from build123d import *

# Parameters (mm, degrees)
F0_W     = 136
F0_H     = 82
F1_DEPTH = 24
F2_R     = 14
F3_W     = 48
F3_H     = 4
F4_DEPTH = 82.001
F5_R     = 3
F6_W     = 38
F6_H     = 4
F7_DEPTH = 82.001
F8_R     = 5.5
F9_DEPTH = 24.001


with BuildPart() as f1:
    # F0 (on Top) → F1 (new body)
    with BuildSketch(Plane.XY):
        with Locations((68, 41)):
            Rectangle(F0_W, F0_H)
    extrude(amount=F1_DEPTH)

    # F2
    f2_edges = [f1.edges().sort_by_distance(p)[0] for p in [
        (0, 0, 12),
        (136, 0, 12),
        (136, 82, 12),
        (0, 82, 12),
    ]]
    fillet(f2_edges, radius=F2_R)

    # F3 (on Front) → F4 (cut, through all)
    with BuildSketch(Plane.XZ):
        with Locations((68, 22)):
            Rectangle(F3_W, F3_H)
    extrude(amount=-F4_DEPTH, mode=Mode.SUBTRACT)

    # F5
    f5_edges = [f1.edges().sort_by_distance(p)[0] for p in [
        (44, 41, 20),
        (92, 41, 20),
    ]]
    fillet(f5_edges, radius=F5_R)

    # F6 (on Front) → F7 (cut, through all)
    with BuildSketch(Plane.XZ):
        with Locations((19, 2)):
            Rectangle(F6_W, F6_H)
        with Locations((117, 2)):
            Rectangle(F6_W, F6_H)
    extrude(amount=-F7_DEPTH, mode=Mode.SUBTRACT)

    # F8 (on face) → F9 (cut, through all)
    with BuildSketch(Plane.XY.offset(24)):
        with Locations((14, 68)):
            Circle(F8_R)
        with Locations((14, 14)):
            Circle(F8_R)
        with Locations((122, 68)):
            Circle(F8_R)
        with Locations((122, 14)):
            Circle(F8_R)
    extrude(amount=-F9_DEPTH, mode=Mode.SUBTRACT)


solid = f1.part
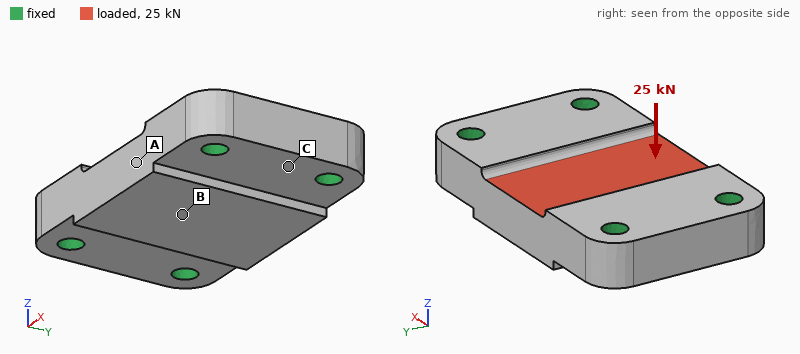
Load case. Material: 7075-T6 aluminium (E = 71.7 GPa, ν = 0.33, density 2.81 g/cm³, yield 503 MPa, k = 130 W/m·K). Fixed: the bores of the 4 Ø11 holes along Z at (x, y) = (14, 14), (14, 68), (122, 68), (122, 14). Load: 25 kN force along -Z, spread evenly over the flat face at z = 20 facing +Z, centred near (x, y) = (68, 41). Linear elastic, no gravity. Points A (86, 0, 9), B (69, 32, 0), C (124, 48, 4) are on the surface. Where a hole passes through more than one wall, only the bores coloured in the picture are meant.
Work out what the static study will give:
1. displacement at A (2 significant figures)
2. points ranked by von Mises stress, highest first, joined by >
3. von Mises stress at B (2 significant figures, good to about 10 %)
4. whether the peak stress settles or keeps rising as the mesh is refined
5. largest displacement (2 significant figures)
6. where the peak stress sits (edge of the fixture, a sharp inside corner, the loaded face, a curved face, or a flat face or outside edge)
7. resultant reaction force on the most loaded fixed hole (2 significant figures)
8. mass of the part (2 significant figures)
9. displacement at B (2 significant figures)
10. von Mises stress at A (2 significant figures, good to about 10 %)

40 µm
B > A > C
39 MPa
keeps rising
51 µm
edge of the fixture
7.2 kN
610 g
46 µm
26 MPa
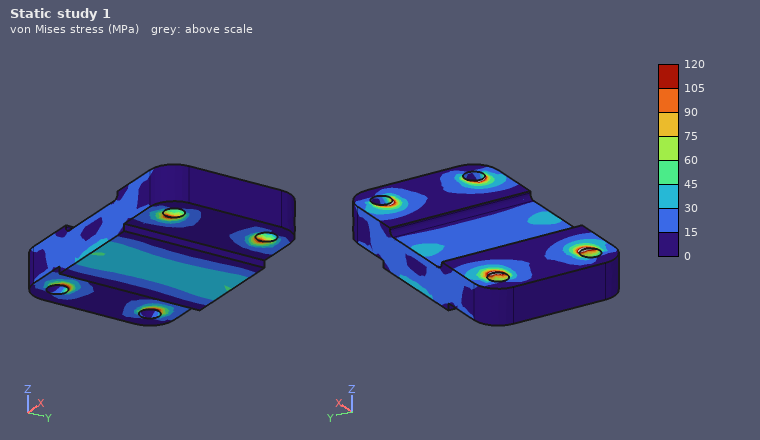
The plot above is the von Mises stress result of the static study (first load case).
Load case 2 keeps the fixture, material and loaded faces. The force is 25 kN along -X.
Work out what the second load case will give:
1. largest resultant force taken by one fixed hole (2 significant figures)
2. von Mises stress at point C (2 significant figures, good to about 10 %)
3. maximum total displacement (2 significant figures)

6.4 kN
3.7 MPa
8.8 µm
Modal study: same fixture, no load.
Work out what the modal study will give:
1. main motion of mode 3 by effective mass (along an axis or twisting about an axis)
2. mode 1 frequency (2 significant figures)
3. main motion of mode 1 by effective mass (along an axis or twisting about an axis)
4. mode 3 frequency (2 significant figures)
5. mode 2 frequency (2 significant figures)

along Y
7400 Hz
along Z
13 kHz
9500 Hz
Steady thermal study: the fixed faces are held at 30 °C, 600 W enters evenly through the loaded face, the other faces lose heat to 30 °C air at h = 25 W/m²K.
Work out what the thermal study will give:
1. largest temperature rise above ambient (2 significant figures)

70 K
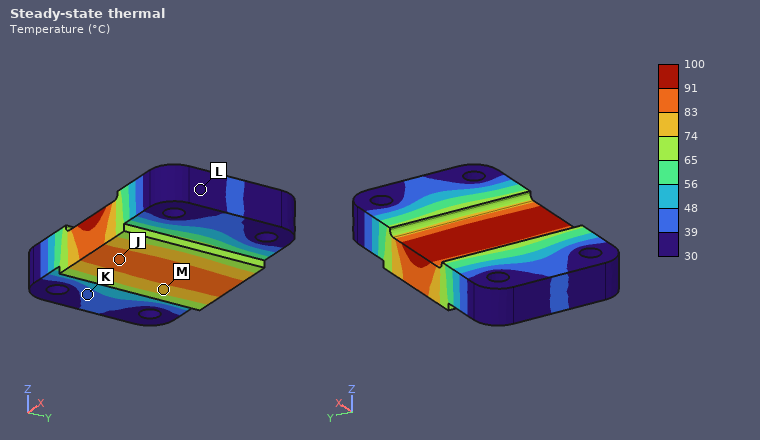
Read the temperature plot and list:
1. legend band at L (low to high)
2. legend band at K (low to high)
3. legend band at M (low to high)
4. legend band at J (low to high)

30 to 39 °C
39 to 48 °C
74 to 83 °C
83 to 91 °C
